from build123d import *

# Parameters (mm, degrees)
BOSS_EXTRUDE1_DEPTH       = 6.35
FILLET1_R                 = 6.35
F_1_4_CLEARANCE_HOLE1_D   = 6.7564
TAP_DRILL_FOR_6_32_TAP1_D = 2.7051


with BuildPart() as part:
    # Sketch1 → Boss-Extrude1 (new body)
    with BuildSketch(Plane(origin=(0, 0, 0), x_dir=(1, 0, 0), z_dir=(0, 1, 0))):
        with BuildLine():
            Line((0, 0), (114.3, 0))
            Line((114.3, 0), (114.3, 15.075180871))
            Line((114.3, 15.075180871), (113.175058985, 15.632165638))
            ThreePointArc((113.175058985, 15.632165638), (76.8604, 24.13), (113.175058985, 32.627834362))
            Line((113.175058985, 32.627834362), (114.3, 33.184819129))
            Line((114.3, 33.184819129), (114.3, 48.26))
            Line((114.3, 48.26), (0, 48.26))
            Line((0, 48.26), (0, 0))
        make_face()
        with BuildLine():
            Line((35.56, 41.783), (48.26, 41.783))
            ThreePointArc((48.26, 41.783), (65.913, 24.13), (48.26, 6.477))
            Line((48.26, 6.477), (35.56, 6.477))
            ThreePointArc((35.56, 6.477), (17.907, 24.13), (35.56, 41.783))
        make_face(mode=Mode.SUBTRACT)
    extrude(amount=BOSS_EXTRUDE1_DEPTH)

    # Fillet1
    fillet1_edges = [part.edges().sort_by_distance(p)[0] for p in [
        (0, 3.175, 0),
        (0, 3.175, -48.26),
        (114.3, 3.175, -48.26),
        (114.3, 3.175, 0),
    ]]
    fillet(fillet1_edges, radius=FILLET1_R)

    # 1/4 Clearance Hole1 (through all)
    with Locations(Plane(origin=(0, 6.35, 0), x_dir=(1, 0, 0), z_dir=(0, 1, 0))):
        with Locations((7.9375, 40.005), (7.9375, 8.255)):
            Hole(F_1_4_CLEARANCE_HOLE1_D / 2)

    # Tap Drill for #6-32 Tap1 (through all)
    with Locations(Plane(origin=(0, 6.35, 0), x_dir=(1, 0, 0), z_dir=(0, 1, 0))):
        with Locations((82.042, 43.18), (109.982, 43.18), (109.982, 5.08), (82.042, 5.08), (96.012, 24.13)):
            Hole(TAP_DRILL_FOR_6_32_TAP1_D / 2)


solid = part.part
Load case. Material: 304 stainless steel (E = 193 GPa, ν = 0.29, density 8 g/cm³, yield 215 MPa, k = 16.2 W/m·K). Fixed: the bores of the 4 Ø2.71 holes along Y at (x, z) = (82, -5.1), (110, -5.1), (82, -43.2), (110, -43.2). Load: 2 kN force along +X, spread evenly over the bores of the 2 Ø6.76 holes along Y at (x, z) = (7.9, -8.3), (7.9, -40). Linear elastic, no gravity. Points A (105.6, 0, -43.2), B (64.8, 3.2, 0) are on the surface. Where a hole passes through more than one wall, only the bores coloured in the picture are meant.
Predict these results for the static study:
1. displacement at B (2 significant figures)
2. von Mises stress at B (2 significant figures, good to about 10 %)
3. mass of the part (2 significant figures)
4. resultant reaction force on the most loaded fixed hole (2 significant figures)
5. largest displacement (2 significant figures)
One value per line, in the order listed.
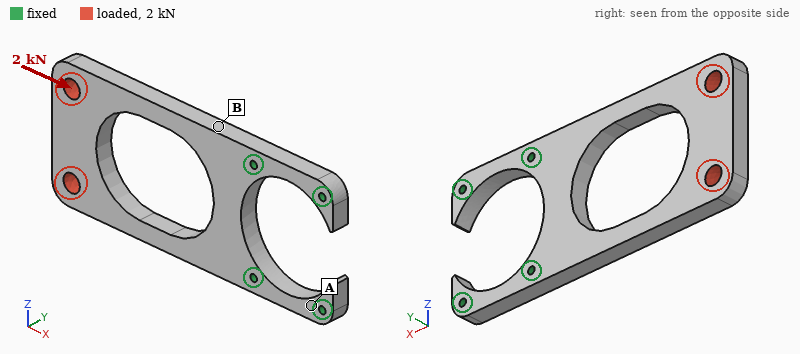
2.3 µm
28 MPa
140 g
970 N
9.8 µm
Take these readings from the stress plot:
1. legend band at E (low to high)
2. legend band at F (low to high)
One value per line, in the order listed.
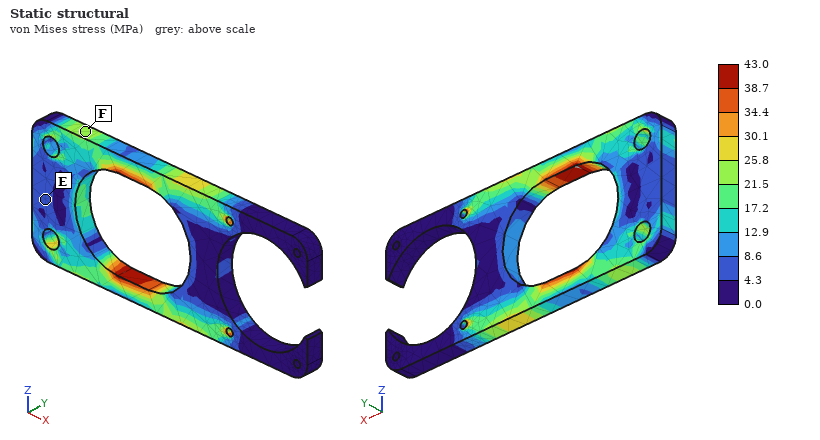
4.3 to 8.6 MPa
21.5 to 25.8 MPa
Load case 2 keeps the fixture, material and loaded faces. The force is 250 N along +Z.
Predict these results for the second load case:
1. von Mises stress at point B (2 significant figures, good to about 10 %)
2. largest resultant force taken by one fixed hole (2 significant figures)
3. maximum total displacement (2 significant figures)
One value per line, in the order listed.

21 MPa
450 N
24 µm
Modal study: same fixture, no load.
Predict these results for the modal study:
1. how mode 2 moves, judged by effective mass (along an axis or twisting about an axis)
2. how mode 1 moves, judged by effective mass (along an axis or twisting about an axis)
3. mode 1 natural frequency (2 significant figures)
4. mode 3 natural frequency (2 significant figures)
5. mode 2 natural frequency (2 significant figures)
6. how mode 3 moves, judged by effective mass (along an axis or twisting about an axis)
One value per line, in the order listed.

twisting about X
along Y
570 Hz
2200 Hz
1900 Hz
along Z
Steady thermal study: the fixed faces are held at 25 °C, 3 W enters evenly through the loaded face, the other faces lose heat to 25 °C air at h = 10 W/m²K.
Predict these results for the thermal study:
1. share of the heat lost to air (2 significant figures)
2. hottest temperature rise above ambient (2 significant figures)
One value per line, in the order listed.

65 %
55 K
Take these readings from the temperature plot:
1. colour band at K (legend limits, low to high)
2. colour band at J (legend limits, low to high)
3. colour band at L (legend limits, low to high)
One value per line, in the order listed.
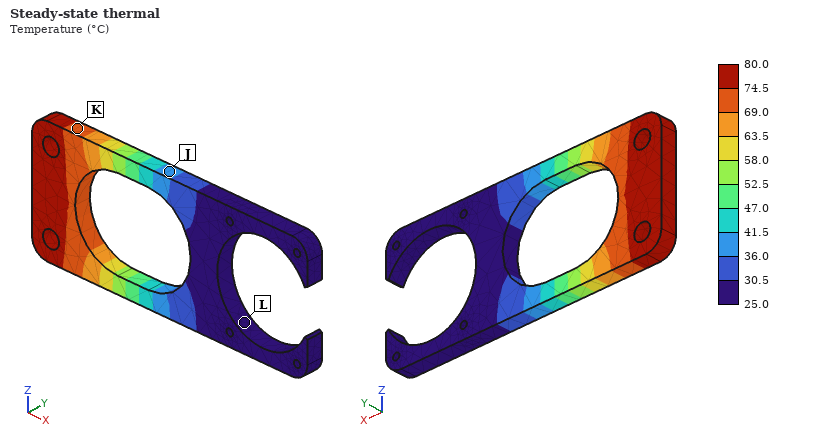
69.0 to 74.5 °C
36.0 to 41.5 °C
25.0 to 30.5 °C
